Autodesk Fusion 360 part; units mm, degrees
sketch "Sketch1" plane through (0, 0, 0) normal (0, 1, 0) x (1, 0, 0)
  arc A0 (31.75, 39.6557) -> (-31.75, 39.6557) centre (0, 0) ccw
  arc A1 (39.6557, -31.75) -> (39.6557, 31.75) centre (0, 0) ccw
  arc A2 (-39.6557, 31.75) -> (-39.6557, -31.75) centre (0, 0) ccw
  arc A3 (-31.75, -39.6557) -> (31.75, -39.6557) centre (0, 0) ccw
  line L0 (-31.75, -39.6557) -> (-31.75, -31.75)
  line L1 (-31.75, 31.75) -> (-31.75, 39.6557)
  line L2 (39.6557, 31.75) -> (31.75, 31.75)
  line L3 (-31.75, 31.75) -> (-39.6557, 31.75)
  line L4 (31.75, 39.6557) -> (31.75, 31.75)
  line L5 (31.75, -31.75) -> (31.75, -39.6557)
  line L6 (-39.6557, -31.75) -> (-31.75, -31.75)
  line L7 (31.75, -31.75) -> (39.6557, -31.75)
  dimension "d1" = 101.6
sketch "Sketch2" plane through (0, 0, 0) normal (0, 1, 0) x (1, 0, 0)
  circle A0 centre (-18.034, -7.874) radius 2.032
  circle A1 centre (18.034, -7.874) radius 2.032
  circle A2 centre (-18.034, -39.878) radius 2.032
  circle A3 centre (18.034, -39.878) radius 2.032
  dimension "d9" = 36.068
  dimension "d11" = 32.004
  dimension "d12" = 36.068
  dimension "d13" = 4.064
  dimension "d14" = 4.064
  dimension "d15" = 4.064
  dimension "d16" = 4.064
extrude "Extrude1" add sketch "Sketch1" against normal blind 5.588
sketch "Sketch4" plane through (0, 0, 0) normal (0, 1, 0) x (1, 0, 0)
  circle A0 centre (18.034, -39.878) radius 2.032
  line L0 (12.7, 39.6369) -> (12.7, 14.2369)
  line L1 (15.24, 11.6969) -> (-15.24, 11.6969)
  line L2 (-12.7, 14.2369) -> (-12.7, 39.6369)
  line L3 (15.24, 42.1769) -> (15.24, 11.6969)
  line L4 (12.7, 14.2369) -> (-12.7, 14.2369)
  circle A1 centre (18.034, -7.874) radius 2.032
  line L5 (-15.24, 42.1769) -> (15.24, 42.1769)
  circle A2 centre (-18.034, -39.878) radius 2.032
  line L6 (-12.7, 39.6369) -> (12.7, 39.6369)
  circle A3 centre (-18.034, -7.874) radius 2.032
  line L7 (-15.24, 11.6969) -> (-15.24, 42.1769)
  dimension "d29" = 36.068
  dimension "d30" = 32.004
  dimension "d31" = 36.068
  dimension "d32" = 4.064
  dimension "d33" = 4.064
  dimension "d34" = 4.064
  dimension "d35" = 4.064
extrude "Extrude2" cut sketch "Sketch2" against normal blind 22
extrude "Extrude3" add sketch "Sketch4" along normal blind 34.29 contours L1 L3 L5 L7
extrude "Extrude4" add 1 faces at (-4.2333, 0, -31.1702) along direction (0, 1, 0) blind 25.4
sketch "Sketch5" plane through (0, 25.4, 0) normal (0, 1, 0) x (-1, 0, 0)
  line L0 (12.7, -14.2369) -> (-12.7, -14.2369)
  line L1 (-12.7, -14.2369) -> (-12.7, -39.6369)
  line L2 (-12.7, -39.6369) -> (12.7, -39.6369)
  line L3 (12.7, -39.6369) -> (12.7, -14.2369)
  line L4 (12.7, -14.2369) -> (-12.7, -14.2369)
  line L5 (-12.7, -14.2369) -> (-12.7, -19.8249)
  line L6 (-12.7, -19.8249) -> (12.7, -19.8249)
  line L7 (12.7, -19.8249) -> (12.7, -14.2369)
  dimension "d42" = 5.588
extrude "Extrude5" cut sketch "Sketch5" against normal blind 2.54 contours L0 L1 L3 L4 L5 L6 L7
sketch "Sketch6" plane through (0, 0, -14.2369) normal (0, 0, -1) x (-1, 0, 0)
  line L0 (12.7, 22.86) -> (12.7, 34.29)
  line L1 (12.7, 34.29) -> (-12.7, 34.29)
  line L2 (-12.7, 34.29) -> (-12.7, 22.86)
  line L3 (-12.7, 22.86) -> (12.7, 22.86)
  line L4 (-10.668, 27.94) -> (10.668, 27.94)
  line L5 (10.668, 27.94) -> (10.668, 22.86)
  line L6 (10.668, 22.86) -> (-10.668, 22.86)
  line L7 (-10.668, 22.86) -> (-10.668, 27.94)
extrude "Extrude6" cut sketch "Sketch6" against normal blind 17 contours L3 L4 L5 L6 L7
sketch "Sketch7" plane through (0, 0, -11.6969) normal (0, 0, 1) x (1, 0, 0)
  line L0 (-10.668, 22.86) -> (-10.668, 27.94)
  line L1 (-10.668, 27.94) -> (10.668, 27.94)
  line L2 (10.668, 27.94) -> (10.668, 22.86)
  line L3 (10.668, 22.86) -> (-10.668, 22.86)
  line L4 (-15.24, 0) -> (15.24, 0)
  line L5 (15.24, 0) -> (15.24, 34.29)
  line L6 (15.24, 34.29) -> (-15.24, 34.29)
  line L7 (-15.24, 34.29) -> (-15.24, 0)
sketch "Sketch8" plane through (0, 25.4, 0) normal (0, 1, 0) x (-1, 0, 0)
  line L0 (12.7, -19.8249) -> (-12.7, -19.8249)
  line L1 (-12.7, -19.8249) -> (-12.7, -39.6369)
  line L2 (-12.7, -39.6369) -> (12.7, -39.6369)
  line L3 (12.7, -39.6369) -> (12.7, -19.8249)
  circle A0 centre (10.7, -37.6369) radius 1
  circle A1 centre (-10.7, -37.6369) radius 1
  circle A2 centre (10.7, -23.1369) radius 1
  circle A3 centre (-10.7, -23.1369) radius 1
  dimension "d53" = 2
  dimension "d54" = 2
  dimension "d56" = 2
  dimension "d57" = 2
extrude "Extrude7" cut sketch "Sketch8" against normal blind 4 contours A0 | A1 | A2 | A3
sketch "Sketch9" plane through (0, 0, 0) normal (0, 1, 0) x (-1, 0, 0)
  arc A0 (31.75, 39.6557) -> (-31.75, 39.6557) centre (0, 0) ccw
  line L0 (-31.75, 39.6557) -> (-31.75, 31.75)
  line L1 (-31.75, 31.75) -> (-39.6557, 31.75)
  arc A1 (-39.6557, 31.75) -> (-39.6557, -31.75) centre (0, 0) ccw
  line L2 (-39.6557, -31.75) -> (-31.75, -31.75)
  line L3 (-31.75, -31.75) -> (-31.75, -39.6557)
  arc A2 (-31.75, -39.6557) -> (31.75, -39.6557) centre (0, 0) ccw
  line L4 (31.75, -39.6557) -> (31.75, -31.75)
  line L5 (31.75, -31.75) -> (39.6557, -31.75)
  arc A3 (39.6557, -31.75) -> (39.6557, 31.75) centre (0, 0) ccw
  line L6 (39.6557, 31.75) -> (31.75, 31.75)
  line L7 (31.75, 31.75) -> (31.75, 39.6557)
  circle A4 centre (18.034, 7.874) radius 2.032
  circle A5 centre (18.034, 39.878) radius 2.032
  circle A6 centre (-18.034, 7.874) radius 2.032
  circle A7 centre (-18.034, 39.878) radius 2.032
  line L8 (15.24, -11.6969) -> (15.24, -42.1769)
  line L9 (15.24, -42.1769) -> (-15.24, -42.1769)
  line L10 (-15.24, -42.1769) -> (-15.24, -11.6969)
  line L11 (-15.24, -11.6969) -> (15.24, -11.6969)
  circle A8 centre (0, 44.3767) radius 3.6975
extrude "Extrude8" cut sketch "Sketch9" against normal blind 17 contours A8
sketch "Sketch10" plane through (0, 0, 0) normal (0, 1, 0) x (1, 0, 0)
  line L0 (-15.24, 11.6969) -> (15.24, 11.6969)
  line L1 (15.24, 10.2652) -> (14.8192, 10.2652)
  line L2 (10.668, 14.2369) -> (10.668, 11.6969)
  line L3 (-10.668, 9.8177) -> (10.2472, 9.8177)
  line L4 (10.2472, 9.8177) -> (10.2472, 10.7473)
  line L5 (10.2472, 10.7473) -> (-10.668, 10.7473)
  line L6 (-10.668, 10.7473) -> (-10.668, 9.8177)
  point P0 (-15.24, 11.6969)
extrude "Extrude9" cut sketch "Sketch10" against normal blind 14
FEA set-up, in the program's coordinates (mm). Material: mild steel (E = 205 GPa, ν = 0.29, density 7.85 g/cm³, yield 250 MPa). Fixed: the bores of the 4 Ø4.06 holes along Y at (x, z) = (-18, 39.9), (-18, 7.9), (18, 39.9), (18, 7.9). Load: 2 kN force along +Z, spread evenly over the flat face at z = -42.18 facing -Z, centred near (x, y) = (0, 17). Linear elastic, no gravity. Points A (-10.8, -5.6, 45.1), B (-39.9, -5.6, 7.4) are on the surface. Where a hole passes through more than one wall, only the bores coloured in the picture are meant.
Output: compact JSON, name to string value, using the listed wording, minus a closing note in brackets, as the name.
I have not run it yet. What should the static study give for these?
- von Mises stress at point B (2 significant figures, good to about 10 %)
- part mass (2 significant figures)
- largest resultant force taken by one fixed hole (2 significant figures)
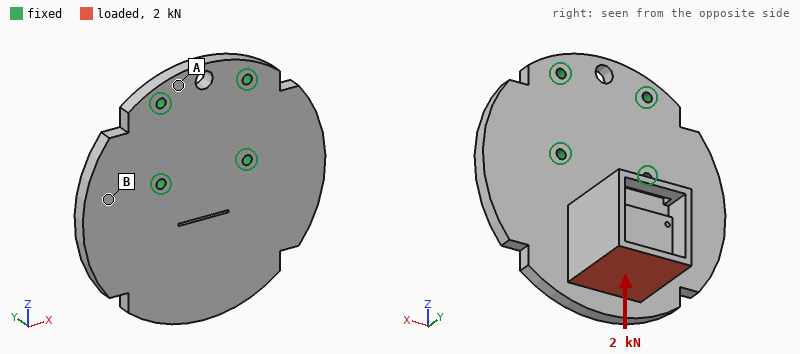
{"von Mises stress at point B": "50 MPa", "part mass": "540 g", "largest resultant force taken by one fixed hole": "910 N"}
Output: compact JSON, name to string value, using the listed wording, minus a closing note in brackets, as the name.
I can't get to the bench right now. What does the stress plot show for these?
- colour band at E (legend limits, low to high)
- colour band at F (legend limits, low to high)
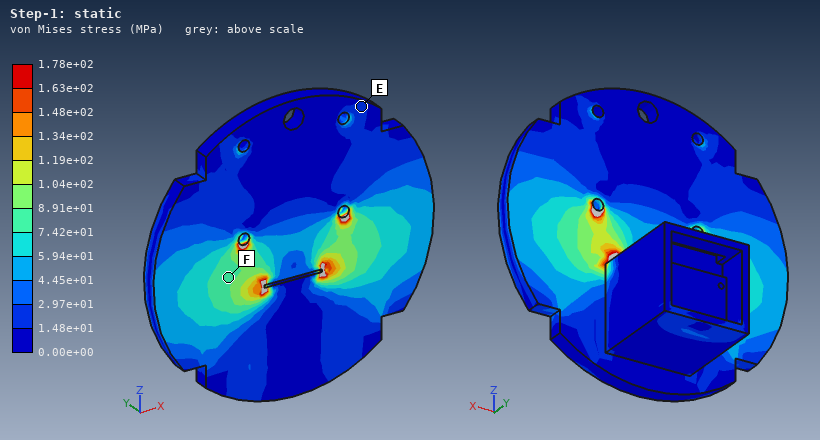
{"colour band at E": "1.48e+01 to 2.97e+01 MPa", "colour band at F": "7.42e+01 to 8.91e+01 MPa"}
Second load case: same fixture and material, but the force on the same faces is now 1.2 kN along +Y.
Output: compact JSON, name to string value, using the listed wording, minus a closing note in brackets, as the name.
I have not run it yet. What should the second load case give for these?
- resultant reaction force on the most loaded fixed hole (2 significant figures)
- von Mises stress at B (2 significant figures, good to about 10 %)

{"resultant reaction force on the most loaded fixed hole": "1.1 kN", "von Mises stress at B": "63 MPa"}
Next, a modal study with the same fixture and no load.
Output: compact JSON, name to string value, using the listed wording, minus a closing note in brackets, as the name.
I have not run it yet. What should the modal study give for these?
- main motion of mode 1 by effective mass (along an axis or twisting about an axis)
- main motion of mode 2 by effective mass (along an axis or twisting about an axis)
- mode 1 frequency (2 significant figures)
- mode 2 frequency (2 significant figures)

{"main motion of mode 1 by effective mass": "along Y", "main motion of mode 2 by effective mass": "along X", "mode 1 frequency": "850 Hz", "mode 2 frequency": "2400 Hz"}
